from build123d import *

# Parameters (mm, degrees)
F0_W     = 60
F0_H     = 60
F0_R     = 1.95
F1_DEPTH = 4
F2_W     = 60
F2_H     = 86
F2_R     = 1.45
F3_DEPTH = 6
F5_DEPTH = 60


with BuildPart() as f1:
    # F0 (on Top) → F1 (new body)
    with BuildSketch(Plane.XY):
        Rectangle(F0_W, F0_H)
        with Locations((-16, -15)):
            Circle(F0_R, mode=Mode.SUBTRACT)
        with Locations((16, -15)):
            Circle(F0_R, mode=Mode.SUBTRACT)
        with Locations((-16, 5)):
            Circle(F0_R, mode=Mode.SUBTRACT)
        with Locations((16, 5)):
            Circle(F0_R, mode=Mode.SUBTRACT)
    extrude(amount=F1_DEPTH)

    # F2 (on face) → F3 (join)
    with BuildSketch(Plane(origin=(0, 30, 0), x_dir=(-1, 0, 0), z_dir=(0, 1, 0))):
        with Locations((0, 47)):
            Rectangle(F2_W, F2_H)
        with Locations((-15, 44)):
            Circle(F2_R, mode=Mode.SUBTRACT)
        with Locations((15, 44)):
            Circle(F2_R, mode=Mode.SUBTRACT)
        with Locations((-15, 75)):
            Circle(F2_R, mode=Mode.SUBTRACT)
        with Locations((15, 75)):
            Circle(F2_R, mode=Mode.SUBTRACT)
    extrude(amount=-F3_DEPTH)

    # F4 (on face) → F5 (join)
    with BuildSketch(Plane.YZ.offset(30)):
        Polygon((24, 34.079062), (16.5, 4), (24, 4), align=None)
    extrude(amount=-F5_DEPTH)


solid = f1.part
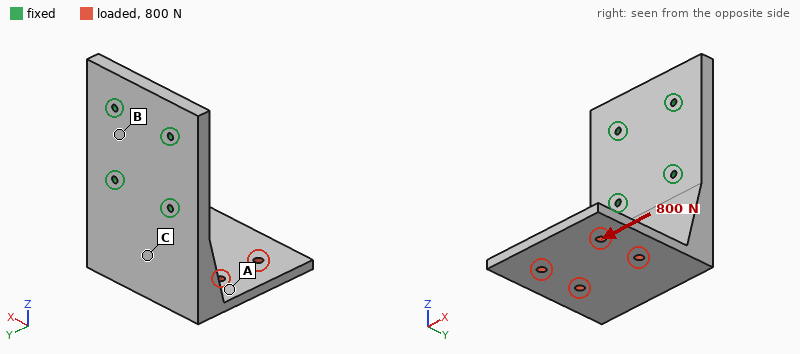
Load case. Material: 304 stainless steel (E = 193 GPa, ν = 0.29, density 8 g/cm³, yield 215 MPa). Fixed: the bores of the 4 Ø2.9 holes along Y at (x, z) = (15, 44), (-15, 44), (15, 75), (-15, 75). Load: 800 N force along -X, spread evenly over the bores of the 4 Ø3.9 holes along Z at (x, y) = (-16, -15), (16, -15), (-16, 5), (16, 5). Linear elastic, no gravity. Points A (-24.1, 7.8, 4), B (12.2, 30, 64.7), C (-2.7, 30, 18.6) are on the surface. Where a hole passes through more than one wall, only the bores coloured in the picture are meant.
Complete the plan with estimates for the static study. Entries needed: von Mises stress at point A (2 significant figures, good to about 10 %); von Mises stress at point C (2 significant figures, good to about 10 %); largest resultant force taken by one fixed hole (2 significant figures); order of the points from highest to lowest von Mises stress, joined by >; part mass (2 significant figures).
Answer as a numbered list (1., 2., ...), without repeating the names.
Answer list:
1. 12 MPa
2. 21 MPa
3. 1.1 kN
4. C > A > B
5. 410 g
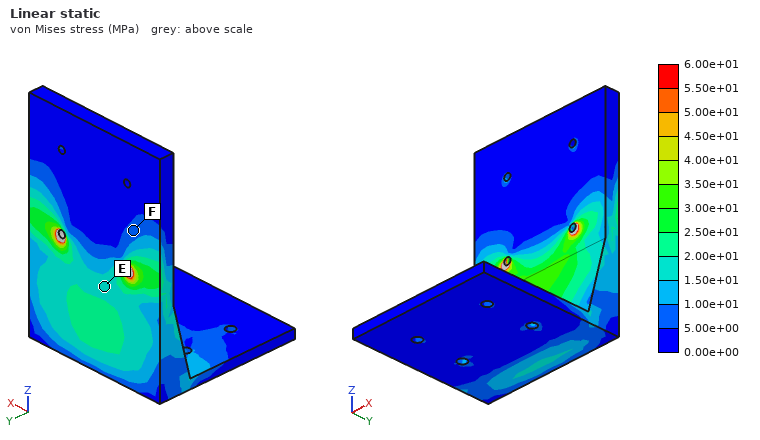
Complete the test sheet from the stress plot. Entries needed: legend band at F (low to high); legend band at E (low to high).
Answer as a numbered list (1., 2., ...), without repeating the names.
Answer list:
1. 5.00e+00 to 1.00e+01 MPa
2. 1.50e+01 to 2.00e+01 MPa
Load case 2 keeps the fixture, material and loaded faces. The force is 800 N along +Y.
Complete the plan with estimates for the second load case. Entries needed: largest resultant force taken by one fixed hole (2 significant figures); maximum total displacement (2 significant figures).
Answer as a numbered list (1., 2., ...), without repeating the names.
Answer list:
1. 650 N
2. 0.18 mm
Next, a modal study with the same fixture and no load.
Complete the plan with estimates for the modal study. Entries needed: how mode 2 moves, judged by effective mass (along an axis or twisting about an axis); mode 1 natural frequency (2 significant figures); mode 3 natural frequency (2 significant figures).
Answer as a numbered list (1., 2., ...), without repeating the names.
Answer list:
1. along Y
2. 830 Hz
3. 1900 Hz
